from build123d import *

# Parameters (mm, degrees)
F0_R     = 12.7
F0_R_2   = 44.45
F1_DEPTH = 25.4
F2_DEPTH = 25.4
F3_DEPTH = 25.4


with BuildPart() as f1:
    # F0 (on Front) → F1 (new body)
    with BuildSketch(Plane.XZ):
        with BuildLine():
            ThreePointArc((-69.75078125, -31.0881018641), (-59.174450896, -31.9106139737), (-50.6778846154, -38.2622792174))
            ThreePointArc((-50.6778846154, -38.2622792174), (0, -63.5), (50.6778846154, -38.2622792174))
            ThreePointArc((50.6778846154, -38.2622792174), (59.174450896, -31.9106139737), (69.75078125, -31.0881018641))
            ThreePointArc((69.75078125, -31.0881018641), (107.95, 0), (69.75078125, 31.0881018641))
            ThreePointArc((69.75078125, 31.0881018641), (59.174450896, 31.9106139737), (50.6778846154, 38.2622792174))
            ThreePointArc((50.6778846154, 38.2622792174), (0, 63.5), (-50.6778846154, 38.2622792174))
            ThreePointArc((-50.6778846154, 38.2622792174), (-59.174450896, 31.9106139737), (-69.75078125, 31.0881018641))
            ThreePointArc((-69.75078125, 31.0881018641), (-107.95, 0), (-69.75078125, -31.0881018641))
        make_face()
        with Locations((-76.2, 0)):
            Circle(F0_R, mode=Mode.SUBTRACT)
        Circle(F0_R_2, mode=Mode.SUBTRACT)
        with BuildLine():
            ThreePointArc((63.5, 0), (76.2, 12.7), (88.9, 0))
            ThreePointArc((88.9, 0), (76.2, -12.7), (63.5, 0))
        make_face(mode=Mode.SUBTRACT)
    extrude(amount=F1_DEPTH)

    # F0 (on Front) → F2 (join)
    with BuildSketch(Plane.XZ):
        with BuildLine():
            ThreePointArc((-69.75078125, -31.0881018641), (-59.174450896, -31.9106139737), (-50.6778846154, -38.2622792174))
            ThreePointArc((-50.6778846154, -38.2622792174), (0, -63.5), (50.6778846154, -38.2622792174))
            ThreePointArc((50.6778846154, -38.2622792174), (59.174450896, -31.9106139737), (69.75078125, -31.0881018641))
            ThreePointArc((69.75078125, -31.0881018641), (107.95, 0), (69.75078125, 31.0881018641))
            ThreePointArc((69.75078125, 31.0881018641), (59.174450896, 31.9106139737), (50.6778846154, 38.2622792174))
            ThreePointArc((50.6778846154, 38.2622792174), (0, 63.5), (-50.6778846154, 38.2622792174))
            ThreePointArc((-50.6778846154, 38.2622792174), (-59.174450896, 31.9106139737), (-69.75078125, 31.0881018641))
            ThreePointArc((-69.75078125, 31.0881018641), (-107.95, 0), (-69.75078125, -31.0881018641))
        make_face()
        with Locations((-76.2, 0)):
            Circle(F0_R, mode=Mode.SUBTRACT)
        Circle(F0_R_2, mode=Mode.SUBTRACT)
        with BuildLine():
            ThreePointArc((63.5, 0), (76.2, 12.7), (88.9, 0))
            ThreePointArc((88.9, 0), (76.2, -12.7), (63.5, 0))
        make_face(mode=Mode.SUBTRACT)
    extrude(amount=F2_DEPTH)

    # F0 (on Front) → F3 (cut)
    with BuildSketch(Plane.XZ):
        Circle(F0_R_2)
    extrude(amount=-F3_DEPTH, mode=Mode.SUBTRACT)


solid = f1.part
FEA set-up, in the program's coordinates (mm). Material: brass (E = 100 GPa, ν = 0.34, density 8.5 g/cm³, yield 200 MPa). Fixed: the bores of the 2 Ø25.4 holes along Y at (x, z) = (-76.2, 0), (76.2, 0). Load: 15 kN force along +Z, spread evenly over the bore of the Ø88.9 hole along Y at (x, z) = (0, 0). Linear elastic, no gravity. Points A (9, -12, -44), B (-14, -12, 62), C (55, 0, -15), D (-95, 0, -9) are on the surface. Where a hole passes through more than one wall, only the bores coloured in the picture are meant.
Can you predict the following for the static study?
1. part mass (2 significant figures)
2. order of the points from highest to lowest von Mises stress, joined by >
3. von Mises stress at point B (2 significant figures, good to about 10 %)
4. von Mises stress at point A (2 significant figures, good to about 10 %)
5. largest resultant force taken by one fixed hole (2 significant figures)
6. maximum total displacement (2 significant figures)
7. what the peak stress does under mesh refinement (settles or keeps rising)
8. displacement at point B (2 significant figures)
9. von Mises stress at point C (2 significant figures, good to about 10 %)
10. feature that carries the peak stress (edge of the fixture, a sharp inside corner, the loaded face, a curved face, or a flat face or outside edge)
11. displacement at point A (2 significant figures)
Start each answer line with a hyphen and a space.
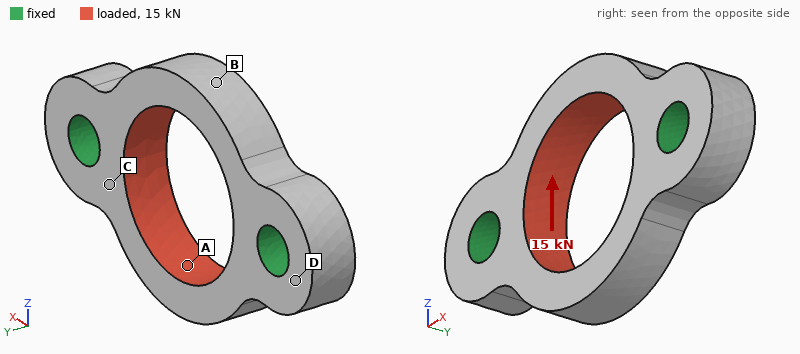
- 2.3 kg
- C > B > A > D
- 6.4 MPa
- 4.3 MPa
- 7.5 kN
- 8.2 µm
- keeps rising
- 7.3 µm
- 8.7 MPa
- edge of the fixture
- 8.0 µm
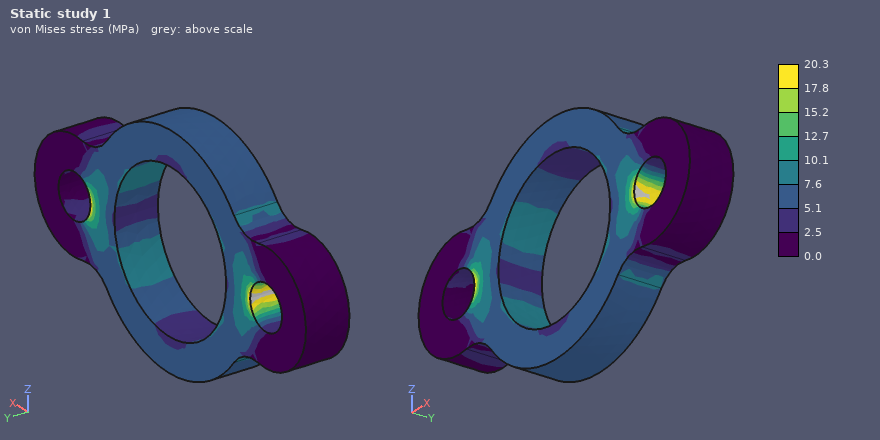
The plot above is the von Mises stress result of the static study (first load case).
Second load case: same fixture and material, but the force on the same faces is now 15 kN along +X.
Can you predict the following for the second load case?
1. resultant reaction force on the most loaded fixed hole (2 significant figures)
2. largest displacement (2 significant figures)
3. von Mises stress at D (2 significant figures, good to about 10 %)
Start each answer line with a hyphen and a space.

- 7.5 kN
- 7.5 µm
- 1.9 MPa
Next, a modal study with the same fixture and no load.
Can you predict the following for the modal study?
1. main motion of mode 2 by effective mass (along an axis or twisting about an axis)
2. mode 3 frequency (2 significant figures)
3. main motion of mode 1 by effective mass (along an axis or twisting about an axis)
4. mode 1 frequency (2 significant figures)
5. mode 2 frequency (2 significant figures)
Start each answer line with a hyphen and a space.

- along Y
- 5600 Hz
- twisting about X
- 2500 Hz
- 2700 Hz
